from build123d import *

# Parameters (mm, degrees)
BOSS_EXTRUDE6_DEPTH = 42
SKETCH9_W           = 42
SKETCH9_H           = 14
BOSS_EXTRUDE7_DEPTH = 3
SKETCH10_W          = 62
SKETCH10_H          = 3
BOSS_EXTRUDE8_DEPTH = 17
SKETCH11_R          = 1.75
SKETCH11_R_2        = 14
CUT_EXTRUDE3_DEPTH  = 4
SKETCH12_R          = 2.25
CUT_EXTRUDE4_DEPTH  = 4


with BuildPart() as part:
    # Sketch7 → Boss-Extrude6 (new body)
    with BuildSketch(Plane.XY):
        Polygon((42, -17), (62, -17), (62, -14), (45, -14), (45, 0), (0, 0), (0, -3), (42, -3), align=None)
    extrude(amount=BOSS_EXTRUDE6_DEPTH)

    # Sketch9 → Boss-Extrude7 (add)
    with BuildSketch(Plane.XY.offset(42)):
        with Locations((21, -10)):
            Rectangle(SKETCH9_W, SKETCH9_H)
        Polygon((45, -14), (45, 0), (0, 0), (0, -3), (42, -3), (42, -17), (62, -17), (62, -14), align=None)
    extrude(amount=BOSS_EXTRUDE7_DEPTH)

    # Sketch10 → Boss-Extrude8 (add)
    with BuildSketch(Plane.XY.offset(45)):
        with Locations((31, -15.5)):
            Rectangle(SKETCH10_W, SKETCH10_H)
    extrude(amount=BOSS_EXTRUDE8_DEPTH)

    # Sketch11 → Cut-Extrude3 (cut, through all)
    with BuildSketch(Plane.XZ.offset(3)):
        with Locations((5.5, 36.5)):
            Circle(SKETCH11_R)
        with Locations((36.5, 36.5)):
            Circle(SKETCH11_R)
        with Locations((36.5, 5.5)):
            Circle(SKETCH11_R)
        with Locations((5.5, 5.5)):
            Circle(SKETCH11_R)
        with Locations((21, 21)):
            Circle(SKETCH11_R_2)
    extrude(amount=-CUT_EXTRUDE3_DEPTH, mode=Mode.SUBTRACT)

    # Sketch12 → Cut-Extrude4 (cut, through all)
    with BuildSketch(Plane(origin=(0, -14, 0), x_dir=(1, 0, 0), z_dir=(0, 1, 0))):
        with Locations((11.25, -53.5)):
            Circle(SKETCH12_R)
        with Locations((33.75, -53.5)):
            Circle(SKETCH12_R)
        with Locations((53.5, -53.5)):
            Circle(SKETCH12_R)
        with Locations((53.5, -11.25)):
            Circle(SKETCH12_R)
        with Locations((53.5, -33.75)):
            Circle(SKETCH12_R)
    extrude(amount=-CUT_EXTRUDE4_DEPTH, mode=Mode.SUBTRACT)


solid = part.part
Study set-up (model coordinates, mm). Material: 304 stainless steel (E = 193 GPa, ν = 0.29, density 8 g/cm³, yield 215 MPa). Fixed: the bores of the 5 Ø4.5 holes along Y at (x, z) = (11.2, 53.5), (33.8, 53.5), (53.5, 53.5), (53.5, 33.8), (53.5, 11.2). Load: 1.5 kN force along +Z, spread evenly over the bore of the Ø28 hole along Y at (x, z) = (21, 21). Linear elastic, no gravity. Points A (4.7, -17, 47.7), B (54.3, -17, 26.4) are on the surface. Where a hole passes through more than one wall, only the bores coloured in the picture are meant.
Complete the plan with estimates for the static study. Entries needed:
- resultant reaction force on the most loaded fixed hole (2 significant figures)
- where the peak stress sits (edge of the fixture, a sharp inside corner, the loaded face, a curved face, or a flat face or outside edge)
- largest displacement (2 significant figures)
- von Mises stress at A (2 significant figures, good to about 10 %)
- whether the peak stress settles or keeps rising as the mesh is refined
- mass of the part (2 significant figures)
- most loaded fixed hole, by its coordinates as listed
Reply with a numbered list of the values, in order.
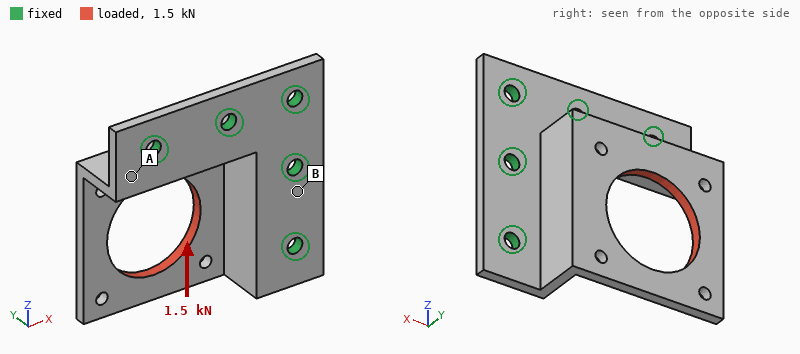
1. 940 N
2. edge of the fixture
3. 93 µm
4. 80 MPa
5. keeps rising
6. 100 g
7. (53.5, 11.2)
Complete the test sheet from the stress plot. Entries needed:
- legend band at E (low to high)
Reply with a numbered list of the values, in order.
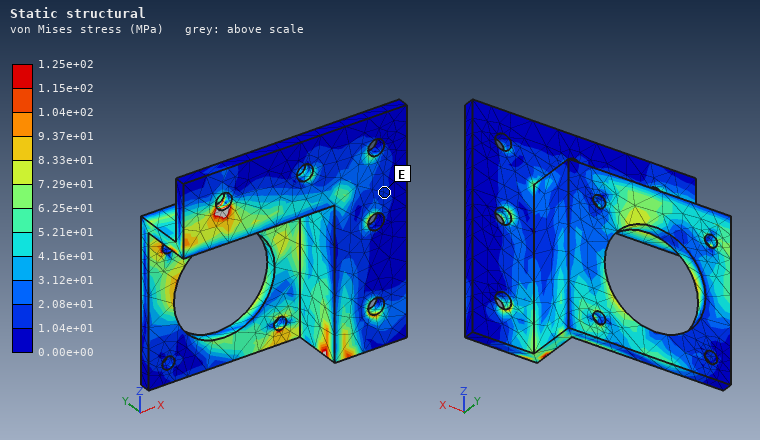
1. 1.04e+01 to 2.08e+01 MPa
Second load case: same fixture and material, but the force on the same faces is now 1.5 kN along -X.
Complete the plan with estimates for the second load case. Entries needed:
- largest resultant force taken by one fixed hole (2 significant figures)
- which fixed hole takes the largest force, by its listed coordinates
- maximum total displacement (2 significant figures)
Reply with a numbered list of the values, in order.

1. 940 N
2. (11.2, 53.5)
3. 93 µm
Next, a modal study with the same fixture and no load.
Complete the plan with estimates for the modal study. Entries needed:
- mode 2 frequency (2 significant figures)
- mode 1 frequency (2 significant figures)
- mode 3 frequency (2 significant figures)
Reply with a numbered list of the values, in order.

1. 3400 Hz
2. 1900 Hz
3. 5900 Hz
